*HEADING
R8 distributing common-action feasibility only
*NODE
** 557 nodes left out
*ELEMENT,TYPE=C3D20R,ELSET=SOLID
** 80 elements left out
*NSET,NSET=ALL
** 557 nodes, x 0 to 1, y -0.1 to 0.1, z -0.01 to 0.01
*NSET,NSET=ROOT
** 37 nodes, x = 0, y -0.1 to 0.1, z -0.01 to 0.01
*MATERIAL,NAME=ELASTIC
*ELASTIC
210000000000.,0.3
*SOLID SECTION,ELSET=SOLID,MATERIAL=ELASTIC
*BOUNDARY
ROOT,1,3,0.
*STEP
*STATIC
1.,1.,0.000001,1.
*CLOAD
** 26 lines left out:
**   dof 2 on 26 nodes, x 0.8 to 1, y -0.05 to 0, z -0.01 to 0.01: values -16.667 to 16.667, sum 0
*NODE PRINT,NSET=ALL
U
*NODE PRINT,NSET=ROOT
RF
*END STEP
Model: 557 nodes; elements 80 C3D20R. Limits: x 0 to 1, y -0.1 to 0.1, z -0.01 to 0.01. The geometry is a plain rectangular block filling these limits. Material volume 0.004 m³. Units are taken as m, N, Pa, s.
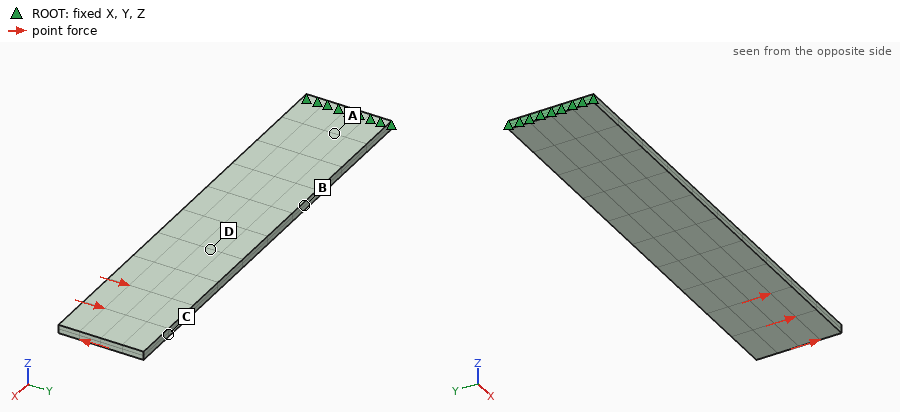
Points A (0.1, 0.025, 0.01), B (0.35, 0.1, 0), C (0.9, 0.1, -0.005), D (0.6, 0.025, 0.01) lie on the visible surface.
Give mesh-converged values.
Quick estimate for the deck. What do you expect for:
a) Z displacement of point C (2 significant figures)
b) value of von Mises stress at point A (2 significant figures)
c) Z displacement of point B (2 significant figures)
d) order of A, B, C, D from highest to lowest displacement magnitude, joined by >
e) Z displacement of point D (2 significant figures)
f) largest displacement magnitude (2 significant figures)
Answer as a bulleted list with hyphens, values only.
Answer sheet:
- 2.0e-06 m
- 61000 Pa
- 7.5e-07 m
- C > B > D > A
- 3.4e-07 m
- 2.1e-06 m
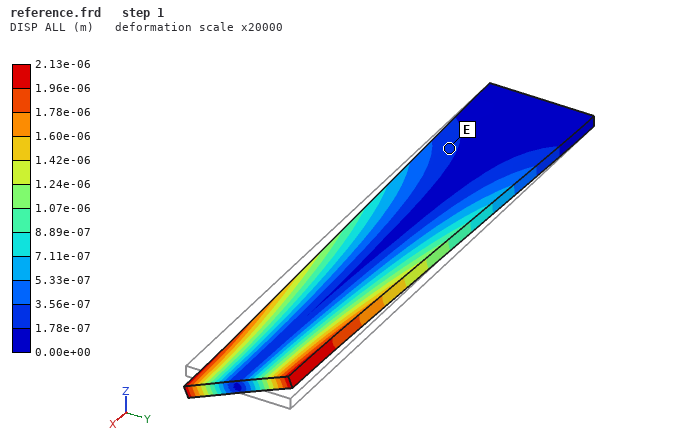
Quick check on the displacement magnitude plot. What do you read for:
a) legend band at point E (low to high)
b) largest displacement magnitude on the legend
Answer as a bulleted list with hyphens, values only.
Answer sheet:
- 1.78e-07 to 3.56e-07 m
- 2.13e-06 m
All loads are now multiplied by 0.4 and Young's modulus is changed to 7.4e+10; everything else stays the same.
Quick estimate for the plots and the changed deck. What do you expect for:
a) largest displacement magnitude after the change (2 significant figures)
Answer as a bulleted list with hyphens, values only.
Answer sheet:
- 2.4e-06 m
